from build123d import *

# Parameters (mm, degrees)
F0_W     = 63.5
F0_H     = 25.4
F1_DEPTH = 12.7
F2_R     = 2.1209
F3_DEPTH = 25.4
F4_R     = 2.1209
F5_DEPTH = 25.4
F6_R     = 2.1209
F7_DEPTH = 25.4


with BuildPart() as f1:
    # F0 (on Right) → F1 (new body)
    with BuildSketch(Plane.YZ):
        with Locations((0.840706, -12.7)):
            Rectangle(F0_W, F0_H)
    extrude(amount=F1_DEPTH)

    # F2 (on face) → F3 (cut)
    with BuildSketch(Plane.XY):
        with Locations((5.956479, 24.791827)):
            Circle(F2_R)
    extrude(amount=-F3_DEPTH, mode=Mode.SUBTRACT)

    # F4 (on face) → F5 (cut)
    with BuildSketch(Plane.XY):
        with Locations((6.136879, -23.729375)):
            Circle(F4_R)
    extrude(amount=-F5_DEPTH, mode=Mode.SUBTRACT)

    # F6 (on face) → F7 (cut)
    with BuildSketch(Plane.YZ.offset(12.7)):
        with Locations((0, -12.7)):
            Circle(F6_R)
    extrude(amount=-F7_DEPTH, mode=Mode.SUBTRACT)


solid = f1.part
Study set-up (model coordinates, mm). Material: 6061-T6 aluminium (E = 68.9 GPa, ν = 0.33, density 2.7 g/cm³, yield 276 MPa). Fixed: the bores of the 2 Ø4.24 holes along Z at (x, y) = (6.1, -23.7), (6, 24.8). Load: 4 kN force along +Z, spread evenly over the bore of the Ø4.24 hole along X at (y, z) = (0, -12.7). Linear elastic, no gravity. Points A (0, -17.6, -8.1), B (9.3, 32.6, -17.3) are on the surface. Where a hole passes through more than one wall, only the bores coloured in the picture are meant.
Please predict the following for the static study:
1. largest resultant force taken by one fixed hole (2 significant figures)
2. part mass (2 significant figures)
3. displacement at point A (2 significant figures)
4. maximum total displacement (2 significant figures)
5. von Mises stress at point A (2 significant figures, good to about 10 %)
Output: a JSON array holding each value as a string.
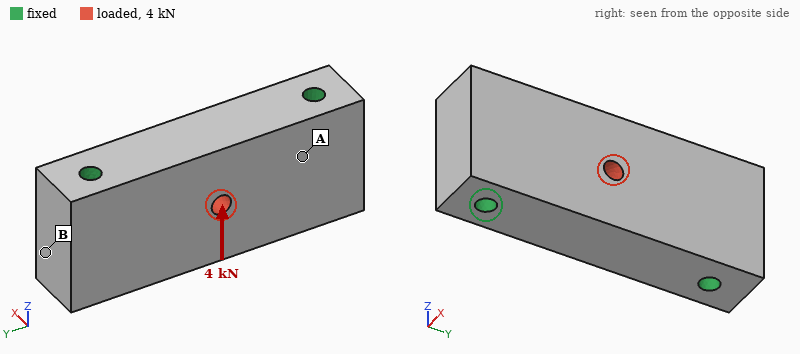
["2.1 kN", "53 g", "1.8 µm", "9.1 µm", "13 MPa"]
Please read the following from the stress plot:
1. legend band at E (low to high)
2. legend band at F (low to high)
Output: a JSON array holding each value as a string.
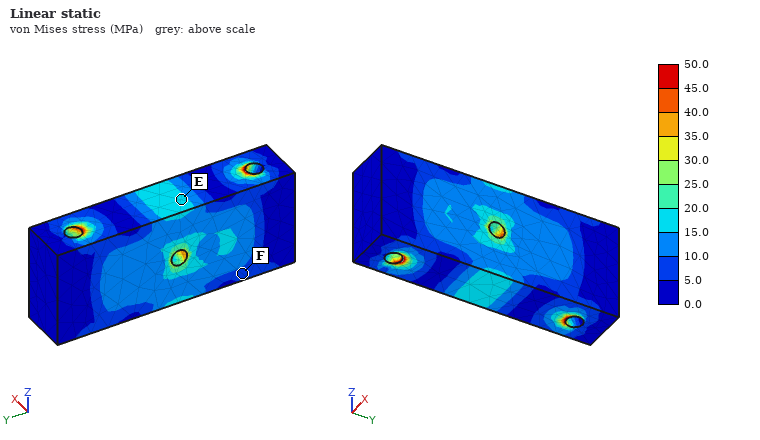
["15.0 to 20.0 MPa", "5.0 to 10.0 MPa"]
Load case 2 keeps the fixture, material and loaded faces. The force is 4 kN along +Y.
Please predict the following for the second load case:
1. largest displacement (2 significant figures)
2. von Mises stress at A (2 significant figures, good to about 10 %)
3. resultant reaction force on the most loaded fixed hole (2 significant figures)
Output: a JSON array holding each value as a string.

["3.6 µm", "5.6 MPa", "2.0 kN"]
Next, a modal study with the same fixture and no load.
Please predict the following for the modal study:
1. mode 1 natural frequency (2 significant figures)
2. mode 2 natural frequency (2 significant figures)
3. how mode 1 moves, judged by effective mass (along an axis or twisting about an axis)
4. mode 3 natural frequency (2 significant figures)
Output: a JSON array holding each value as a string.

["18 kHz", "26 kHz", "along X", "27 kHz"]
